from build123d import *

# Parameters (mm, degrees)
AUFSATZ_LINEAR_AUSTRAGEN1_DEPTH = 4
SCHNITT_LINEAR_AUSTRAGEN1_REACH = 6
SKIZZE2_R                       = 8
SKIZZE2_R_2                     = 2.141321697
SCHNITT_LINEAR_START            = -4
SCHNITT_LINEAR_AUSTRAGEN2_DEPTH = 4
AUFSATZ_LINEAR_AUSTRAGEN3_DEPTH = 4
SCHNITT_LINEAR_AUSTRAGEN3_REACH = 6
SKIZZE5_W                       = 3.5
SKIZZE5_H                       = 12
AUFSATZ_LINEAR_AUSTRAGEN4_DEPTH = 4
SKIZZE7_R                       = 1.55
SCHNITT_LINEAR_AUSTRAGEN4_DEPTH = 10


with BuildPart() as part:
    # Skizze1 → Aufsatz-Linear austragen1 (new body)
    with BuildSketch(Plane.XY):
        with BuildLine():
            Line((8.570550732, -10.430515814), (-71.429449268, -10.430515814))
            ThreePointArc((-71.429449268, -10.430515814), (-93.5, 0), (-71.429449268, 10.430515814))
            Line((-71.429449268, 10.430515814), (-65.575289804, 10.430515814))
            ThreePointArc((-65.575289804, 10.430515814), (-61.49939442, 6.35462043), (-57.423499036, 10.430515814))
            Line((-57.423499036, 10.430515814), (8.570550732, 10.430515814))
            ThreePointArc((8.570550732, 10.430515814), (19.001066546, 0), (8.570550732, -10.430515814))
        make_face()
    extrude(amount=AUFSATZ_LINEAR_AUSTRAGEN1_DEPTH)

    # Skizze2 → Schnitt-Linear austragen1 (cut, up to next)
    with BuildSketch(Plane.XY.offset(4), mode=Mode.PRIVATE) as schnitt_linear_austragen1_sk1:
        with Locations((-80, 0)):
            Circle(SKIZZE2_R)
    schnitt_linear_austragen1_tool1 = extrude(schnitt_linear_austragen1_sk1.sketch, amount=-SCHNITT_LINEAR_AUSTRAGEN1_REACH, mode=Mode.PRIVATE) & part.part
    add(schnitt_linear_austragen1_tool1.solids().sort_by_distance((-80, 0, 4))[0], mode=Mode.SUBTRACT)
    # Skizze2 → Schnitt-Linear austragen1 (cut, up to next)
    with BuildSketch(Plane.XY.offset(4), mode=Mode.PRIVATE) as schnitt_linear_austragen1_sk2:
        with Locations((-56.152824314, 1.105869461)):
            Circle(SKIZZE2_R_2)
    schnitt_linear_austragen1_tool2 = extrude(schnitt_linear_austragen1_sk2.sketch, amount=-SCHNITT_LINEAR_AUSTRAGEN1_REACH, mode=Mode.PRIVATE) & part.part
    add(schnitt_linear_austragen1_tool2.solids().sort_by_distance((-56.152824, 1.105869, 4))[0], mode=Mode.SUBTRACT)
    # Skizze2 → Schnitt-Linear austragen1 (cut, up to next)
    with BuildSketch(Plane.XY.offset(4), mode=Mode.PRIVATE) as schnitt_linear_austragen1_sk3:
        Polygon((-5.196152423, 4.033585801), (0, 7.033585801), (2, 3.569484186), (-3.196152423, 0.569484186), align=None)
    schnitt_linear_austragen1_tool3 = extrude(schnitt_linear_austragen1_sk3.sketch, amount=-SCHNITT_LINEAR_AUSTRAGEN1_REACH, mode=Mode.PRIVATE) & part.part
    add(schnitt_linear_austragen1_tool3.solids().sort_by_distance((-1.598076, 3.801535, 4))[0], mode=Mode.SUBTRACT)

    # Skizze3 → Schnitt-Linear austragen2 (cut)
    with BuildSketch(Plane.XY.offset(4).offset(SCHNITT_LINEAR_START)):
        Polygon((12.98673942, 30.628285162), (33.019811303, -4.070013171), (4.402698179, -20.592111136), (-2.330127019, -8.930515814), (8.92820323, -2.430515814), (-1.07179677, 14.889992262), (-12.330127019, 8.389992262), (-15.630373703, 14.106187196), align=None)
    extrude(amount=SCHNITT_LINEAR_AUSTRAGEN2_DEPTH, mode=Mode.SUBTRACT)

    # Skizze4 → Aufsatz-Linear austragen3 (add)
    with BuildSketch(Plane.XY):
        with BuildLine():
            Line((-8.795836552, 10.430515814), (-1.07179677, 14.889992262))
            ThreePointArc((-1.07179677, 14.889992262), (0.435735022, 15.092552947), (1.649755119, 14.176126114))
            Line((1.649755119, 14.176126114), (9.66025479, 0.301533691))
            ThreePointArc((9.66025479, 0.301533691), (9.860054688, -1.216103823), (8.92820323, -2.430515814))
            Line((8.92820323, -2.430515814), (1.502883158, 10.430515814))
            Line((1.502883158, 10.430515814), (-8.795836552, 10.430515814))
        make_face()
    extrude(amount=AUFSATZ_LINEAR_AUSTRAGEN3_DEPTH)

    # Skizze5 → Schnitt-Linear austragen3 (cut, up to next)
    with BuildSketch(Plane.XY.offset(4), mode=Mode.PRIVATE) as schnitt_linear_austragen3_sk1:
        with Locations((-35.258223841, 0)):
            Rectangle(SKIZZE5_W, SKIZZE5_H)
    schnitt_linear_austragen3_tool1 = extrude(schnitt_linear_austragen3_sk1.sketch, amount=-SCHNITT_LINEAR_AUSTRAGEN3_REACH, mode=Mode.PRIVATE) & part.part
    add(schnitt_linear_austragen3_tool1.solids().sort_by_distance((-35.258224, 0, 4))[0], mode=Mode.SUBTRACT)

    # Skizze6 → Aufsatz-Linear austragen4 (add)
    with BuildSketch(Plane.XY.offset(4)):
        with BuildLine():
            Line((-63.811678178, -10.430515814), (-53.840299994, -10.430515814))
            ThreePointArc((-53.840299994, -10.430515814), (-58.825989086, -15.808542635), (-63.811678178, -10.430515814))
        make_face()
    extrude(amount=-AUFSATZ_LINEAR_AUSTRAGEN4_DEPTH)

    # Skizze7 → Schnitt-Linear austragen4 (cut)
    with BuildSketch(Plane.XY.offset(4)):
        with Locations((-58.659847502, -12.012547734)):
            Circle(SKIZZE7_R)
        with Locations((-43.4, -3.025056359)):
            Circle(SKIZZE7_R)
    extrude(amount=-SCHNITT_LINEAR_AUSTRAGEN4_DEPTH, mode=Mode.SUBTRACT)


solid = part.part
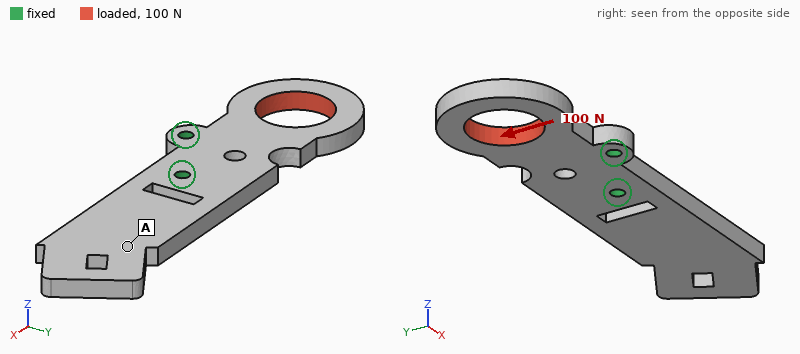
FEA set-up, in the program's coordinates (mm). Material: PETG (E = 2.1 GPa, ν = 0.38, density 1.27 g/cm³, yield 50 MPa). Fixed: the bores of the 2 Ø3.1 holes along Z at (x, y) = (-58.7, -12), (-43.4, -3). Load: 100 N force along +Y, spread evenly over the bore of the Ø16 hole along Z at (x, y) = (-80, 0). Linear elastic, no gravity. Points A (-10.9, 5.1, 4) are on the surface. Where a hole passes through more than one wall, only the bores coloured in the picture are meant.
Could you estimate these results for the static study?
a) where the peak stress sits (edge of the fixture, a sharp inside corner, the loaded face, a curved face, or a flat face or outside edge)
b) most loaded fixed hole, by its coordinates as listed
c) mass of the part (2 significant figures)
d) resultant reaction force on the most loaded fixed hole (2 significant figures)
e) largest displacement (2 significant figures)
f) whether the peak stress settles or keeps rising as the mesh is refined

edge of the fixture
(-58.7, -12)
9.4 g
190 N
0.47 mm
keeps rising
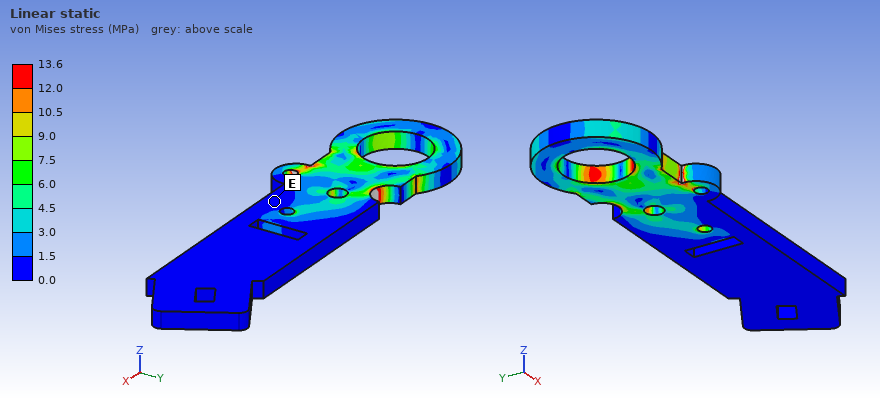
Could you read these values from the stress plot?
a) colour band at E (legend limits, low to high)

0.0 to 1.5 MPa
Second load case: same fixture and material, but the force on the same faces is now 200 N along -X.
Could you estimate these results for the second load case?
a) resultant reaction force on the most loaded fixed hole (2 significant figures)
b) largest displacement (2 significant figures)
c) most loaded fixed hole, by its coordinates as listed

160 N
0.19 mm
(-43.4, -3)
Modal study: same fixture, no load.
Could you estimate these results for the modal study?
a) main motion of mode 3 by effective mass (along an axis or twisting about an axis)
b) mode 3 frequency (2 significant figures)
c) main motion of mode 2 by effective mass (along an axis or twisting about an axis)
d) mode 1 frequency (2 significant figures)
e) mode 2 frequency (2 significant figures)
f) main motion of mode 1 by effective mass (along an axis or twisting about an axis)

along Y
1000 Hz
along Z
260 Hz
590 Hz
along Z
